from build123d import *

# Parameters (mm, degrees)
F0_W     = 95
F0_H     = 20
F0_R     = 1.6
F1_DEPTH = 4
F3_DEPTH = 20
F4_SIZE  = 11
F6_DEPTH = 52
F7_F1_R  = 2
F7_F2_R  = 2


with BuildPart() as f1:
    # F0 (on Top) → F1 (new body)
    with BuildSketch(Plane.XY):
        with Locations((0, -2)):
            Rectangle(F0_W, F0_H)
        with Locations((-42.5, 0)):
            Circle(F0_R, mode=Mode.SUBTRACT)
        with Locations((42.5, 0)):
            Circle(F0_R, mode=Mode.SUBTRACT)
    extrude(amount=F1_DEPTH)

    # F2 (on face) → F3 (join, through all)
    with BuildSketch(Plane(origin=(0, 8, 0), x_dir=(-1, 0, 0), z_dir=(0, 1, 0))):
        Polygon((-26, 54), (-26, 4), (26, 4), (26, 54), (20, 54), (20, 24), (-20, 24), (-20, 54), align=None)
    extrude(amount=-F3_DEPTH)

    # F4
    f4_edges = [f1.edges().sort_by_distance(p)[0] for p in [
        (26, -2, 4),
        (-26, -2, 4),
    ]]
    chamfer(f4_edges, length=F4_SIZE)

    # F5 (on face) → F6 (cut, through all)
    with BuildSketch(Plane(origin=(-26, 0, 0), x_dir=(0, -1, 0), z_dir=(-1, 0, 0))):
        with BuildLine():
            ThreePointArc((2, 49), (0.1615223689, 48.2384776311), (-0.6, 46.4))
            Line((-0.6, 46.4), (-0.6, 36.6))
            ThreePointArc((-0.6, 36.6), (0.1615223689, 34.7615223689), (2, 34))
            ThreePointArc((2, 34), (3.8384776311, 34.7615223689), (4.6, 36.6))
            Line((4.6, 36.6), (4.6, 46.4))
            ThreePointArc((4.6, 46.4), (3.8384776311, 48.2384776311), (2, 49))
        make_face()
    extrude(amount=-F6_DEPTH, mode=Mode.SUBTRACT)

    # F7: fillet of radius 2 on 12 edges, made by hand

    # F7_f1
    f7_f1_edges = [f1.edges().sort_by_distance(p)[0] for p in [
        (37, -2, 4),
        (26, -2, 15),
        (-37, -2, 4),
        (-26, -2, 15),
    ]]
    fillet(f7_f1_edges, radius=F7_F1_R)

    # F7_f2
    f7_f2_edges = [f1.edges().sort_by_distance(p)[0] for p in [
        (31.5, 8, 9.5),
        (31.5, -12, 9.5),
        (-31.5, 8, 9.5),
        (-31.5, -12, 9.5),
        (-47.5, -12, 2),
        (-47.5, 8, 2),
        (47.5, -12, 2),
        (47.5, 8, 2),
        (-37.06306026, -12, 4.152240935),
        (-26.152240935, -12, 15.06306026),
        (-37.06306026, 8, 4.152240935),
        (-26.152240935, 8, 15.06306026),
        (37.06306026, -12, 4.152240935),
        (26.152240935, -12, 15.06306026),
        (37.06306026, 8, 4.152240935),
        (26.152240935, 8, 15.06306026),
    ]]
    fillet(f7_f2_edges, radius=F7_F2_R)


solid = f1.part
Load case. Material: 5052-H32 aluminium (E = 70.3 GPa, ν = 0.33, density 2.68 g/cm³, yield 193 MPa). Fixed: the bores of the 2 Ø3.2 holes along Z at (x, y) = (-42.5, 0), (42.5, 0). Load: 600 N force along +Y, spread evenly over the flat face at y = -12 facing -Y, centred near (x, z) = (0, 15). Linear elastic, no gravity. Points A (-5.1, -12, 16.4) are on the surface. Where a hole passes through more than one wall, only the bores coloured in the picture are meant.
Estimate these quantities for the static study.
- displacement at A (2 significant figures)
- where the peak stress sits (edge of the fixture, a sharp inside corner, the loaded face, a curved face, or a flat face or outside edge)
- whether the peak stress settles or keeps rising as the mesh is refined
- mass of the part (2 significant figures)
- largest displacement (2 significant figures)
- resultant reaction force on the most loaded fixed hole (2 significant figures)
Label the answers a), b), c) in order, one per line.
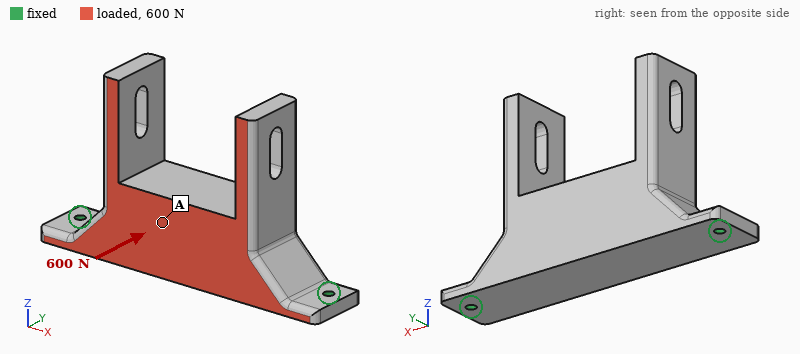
a) 0.063 mm
b) edge of the fixture
c) keeps rising
d) 99 g
e) 0.17 mm
f) 320 N
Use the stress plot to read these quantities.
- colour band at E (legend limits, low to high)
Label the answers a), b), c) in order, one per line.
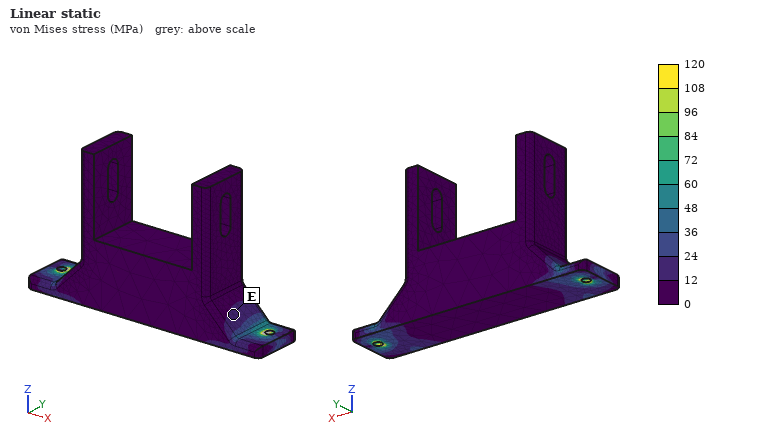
a) 12 to 24 MPa
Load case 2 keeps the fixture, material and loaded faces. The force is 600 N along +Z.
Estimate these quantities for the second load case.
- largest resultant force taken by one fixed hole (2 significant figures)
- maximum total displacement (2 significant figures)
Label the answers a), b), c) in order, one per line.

a) 400 N
b) 0.15 mm
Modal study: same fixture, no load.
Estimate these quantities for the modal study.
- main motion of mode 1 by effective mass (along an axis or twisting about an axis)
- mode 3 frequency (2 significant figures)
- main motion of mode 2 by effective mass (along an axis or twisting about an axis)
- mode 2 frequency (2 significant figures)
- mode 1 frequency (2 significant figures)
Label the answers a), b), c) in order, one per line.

a) along Y
b) 4400 Hz
c) along X
d) 4200 Hz
e) 1300 Hz
